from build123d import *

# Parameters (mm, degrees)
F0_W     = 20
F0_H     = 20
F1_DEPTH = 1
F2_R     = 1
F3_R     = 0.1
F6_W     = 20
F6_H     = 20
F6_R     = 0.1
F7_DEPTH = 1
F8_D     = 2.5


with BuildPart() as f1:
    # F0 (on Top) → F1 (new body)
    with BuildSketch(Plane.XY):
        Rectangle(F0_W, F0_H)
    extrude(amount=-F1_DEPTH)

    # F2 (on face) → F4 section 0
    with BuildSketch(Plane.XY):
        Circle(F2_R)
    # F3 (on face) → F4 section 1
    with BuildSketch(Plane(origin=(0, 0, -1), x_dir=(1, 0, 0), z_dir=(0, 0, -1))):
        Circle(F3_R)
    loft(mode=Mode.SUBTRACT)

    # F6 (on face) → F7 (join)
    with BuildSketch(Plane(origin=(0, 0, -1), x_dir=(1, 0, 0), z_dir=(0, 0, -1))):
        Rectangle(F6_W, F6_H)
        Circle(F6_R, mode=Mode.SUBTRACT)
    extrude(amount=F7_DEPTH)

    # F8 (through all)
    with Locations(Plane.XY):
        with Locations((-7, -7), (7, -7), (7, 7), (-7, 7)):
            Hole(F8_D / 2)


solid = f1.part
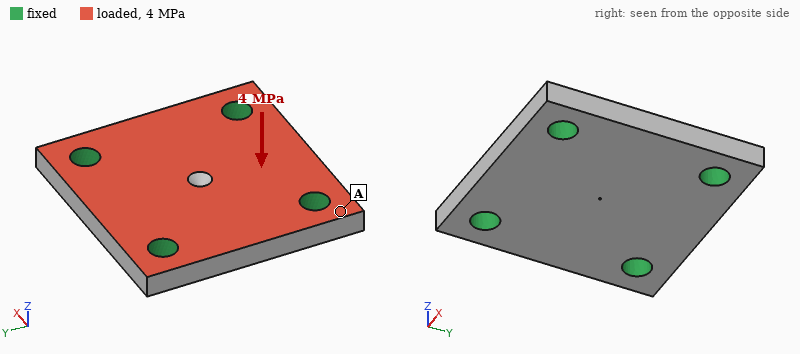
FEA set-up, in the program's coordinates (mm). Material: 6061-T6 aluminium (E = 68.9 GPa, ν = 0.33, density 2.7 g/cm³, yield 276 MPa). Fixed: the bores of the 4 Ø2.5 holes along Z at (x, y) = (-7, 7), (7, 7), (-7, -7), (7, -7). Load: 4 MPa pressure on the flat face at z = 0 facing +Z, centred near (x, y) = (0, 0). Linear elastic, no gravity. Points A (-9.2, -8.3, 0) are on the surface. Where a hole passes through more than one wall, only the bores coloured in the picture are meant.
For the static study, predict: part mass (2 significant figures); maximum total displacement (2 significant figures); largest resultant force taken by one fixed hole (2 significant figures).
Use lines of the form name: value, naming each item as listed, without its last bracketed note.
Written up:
part mass: 2.1 g
maximum total displacement: 17 µm
largest resultant force taken by one fixed hole: 380 N
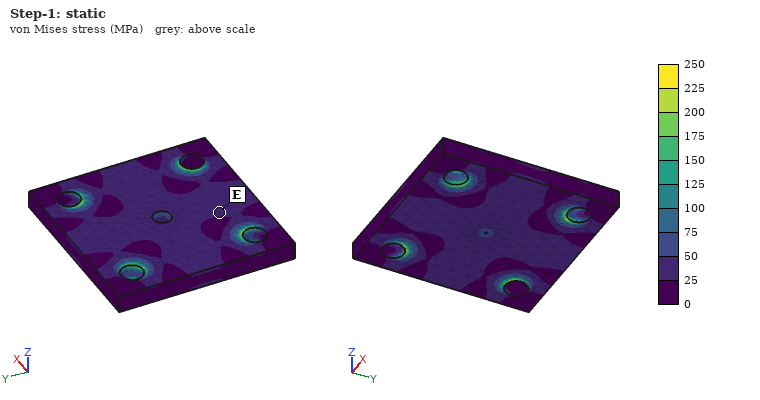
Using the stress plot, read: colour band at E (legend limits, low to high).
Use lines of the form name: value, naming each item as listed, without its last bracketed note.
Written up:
colour band at E: 25 to 50 MPa
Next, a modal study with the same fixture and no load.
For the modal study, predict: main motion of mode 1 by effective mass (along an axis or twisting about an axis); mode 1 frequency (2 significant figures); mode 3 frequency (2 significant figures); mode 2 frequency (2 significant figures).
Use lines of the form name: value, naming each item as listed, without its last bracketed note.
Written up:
main motion of mode 1 by effective mass: along Z
mode 1 frequency: 41 kHz
mode 3 frequency: 60 kHz
mode 2 frequency: 60 kHz
